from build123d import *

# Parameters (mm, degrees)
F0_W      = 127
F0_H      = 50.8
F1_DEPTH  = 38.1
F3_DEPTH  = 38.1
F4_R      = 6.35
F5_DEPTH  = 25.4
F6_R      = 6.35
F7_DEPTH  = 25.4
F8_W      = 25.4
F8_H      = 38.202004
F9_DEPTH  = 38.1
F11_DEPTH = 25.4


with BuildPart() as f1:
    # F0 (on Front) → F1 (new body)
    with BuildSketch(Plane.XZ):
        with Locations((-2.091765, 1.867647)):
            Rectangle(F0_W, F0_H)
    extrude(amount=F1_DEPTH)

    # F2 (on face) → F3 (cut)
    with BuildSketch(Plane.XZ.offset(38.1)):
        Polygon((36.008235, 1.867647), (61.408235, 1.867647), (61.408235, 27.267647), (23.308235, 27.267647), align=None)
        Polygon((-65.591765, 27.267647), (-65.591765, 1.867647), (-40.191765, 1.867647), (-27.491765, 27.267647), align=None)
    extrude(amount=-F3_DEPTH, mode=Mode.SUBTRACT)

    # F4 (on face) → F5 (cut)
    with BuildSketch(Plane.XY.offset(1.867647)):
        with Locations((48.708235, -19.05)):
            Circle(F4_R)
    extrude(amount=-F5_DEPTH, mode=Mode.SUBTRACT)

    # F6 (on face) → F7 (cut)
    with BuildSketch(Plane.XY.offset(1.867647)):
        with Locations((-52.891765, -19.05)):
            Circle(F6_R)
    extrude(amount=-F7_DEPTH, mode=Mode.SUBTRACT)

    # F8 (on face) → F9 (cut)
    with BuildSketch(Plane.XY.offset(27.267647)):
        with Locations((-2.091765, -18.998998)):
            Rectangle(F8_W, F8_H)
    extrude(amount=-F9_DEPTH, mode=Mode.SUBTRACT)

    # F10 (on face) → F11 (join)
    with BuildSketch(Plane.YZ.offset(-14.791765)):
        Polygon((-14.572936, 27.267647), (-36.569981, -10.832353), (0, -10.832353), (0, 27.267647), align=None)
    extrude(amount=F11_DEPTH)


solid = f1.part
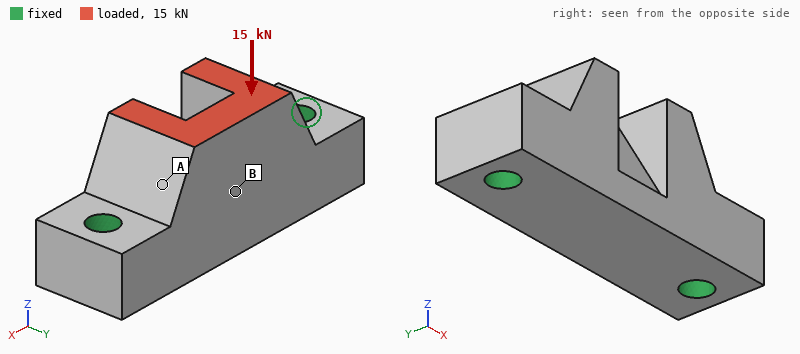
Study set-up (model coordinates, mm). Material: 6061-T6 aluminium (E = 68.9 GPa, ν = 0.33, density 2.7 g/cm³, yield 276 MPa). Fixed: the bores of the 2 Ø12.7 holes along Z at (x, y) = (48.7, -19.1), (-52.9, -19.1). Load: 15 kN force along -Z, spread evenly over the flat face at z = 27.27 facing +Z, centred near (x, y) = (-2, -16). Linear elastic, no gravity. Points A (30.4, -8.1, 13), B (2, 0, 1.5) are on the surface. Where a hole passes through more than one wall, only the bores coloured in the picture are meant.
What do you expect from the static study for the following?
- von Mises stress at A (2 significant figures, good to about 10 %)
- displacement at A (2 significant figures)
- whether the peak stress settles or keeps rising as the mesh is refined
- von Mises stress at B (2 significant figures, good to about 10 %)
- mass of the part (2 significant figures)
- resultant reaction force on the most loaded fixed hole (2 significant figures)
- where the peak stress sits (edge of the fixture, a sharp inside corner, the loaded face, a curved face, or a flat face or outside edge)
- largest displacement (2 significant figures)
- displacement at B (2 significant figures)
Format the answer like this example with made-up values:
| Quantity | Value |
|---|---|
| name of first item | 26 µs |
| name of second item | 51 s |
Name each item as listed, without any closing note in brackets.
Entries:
| Quantity | Value |
|---|---|
| von Mises stress at A | 15 MPa |
| displacement at A | 12 µm |
| whether the peak stress settles or keeps rising as the mesh is refined | keeps rising |
| von Mises stress at B | 5.3 MPa |
| mass of the part | 450 g |
| resultant reaction force on the most loaded fixed hole | 8.0 kN |
| where the peak stress sits | edge of the fixture |
| largest displacement | 25 µm |
| displacement at B | 19 µm |
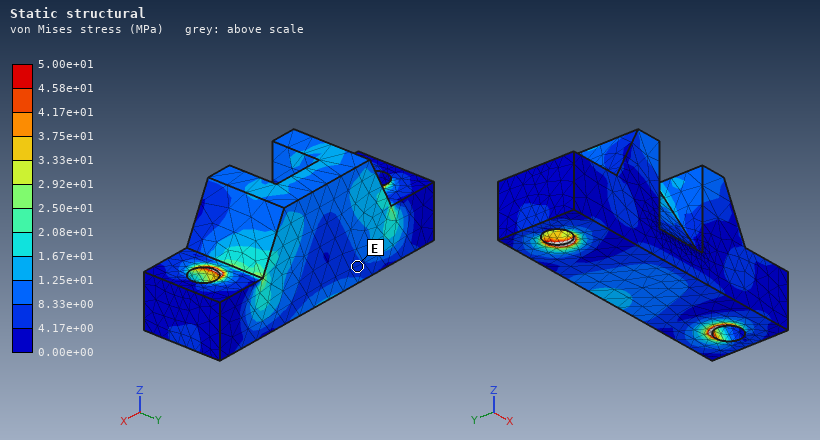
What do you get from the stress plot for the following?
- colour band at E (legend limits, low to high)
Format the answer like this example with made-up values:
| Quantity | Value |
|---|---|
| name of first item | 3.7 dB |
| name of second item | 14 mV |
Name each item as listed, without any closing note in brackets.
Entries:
| Quantity | Value |
|---|---|
| colour band at E | 4.17e+00 to 8.33e+00 MPa |
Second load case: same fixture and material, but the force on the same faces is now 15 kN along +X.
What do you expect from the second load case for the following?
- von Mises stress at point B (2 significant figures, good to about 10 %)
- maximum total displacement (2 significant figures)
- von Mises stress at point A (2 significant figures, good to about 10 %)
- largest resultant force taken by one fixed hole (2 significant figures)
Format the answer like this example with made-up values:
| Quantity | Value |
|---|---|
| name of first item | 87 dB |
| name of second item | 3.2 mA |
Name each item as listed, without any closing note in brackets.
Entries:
| Quantity | Value |
|---|---|
| von Mises stress at point B | 5.5 MPa |
| maximum total displacement | 29 µm |
| von Mises stress at point A | 21 MPa |
| largest resultant force taken by one fixed hole | 9.8 kN |
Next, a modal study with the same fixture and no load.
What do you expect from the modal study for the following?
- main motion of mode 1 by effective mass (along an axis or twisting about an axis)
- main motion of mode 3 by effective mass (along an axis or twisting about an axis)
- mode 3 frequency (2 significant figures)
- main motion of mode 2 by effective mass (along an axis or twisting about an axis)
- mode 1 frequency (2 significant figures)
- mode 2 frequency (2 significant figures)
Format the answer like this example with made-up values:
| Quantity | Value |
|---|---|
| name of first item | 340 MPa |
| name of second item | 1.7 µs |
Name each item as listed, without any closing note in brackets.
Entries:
| Quantity | Value |
|---|---|
| main motion of mode 1 by effective mass | along Y |
| main motion of mode 3 by effective mass | along Y |
| mode 3 frequency | 11 kHz |
| main motion of mode 2 by effective mass | along Z |
| mode 1 frequency | 6500 Hz |
| mode 2 frequency | 9600 Hz |
